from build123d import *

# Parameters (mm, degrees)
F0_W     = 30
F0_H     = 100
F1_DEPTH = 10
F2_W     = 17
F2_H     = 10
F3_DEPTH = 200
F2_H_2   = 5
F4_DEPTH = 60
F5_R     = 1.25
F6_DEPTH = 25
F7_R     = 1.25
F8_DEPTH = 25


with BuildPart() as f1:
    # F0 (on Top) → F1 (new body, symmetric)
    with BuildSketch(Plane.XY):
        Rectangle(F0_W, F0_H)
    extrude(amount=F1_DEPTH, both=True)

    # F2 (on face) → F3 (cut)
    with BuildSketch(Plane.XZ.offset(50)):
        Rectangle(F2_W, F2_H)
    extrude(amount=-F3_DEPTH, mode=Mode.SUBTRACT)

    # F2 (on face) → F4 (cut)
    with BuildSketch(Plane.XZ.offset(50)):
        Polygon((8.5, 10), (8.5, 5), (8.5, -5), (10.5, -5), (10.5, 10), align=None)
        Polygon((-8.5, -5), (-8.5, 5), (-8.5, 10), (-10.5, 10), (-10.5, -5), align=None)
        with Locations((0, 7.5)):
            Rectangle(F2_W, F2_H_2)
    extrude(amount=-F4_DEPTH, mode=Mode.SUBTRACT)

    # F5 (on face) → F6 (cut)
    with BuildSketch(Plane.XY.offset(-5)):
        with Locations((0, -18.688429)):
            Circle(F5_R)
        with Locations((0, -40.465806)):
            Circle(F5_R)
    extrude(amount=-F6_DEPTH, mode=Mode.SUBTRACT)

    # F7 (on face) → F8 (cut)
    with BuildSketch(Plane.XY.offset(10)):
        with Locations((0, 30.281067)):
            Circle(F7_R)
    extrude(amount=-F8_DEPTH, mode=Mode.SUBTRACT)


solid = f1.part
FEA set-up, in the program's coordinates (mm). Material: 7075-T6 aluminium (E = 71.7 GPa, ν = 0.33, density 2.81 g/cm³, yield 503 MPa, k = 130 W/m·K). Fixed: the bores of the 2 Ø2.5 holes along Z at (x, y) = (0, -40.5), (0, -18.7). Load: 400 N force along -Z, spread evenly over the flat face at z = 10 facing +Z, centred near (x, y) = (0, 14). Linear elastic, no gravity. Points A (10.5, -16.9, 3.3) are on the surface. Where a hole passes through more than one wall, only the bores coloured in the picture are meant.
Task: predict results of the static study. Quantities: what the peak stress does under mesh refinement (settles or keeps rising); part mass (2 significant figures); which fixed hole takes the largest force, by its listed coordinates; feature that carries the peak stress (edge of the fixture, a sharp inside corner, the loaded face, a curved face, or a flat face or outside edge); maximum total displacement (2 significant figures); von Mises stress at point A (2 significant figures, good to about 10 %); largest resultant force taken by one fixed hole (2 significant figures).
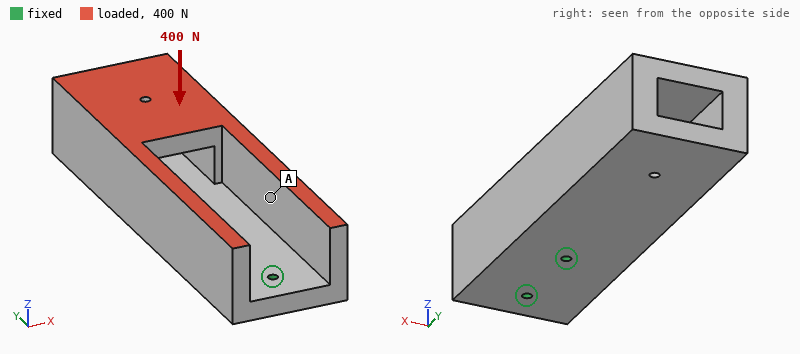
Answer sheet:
keeps rising
96 g
(0, -18.7)
edge of the fixture
94 µm
5.6 MPa
880 N
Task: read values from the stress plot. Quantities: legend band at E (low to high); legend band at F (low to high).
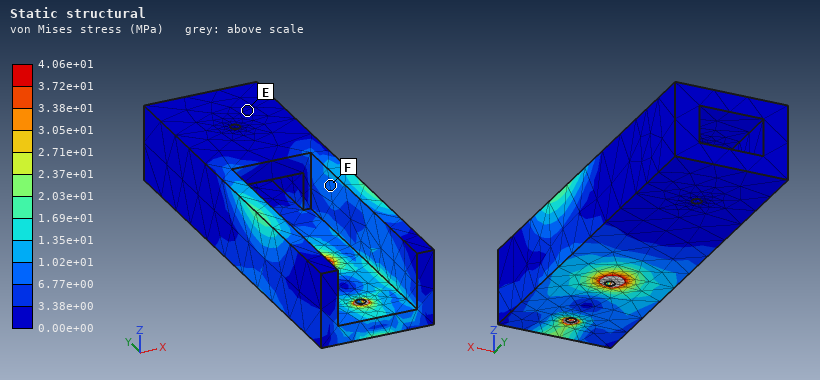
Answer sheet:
0.00e+00 to 3.38e+00 MPa
6.77e+00 to 1.02e+01 MPa
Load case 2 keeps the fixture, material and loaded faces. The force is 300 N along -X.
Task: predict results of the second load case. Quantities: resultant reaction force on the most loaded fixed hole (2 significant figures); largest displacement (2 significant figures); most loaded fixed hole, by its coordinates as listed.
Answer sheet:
720 N
58 µm
(0, -18.7)
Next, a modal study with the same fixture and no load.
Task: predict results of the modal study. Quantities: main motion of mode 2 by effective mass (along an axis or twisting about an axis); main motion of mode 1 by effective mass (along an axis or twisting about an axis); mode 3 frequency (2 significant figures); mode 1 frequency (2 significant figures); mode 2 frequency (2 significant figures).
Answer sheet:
along X
along Z
2800 Hz
1400 Hz
2000 Hz
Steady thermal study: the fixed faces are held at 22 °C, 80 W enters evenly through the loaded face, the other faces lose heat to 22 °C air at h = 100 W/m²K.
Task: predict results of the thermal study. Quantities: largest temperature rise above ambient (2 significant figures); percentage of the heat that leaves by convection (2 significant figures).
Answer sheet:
56 K
49 %
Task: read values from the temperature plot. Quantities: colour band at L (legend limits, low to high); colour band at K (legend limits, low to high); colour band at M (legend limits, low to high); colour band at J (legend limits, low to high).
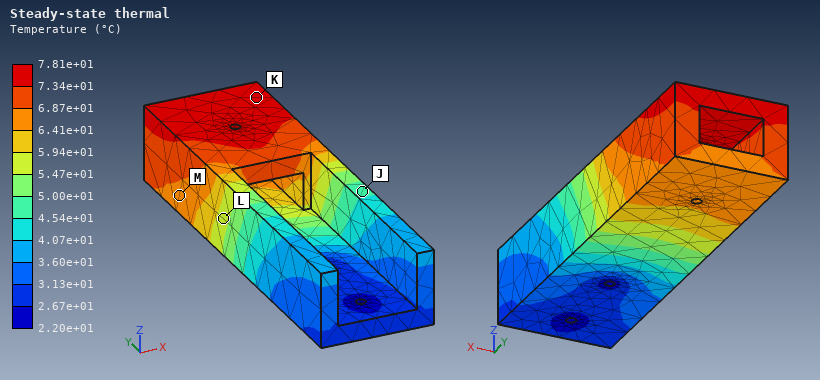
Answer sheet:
5.47e+01 to 5.94e+01 °C
7.34e+01 to 7.81e+01 °C
6.41e+01 to 6.87e+01 °C
4.54e+01 to 5.00e+01 °C
